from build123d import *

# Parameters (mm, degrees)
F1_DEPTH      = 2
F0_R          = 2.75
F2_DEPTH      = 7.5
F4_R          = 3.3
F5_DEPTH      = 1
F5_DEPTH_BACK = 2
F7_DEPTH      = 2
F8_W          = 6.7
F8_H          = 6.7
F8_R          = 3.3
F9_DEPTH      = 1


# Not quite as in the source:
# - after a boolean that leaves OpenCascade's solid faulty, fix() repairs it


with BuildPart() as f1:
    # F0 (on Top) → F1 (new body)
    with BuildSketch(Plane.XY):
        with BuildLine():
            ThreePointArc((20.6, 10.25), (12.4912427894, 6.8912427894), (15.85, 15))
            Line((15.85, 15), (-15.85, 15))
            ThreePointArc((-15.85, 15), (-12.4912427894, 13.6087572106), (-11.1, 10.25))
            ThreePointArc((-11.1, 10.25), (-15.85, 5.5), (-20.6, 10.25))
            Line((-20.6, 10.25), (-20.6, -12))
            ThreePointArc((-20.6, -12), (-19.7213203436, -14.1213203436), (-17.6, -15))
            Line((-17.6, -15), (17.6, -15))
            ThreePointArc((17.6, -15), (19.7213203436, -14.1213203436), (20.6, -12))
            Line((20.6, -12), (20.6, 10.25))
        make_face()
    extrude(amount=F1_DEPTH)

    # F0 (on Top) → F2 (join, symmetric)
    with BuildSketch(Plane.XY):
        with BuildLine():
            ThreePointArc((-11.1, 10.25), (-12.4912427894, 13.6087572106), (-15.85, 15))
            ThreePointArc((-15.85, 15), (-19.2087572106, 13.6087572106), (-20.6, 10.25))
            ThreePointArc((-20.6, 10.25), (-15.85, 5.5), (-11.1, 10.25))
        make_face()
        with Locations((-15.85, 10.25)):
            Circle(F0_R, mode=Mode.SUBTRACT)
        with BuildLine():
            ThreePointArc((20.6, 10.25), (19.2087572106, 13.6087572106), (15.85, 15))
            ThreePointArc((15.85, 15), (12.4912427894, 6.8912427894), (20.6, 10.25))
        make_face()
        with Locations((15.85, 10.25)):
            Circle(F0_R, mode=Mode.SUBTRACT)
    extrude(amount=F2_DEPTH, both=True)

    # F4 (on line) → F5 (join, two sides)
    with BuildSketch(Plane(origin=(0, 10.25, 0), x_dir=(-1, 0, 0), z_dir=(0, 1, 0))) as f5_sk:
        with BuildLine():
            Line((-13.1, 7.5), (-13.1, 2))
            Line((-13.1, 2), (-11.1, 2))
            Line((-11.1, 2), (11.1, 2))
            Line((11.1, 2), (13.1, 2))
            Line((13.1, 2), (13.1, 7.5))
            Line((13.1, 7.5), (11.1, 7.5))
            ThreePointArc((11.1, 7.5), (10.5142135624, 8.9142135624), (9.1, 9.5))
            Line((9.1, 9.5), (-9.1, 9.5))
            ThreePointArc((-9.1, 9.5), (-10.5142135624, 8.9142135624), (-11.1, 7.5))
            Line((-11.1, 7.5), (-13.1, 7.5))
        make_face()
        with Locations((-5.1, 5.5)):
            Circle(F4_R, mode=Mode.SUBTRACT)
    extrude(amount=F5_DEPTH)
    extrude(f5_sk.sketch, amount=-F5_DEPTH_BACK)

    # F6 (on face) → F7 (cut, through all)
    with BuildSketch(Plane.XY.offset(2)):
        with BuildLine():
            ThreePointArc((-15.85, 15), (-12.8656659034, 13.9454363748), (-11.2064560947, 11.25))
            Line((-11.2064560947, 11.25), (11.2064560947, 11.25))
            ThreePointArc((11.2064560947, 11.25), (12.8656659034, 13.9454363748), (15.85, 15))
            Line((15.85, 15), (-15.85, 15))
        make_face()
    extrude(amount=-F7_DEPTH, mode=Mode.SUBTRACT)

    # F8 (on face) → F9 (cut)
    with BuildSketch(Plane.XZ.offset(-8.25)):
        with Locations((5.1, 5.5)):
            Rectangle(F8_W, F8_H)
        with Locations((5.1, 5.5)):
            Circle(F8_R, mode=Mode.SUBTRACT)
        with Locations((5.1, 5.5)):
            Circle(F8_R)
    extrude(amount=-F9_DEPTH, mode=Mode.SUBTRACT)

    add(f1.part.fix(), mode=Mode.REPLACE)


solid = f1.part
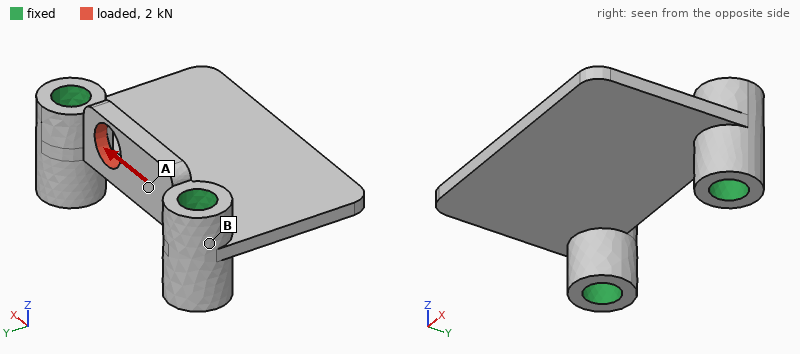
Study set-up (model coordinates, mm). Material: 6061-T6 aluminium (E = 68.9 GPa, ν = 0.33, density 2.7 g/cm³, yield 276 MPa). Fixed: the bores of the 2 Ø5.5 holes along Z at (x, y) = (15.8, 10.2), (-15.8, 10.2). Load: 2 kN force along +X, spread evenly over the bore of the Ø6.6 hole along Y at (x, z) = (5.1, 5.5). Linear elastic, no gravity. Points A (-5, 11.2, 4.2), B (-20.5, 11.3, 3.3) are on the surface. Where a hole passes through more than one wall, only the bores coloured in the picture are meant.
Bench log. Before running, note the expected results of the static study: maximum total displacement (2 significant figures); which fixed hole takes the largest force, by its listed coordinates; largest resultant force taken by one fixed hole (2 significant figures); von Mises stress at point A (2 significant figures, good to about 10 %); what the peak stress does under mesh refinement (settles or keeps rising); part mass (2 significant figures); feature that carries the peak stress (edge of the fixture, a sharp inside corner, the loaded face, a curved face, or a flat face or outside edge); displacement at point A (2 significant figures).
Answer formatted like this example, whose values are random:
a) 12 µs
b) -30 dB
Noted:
a) 15 µm
b) (15.8, 10.2)
c) 1.2 kN
d) 33 MPa
e) keeps rising
f) 10 g
g) a sharp inside corner
h) 3.6 µm
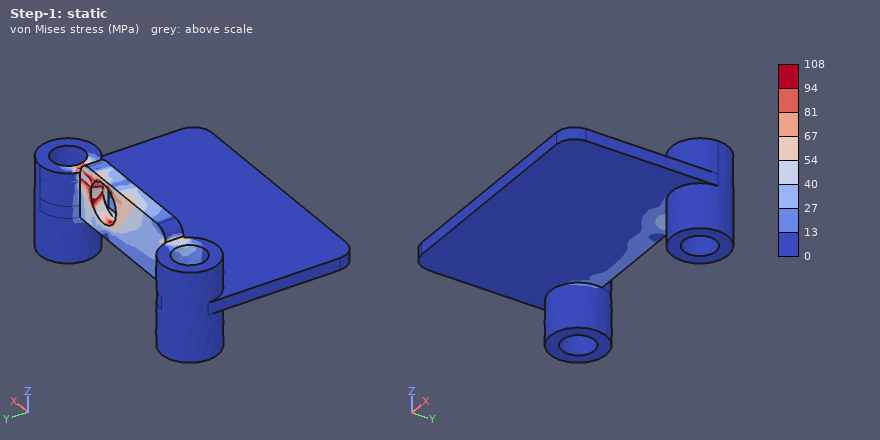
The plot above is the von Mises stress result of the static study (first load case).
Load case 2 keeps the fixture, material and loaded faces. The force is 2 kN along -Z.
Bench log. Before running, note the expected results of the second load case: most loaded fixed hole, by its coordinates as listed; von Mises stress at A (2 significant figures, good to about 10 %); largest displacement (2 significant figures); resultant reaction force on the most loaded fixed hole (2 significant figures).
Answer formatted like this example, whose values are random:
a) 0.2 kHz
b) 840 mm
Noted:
a) (15.8, 10.2)
b) 83 MPa
c) 60 µm
d) 1.3 kN
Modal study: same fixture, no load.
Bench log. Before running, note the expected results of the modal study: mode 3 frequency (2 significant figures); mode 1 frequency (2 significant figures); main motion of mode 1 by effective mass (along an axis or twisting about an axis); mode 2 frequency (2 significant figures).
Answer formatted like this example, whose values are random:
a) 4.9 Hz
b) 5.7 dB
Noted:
a) 10 kHz
b) 3200 Hz
c) along Z
d) 5600 Hz
